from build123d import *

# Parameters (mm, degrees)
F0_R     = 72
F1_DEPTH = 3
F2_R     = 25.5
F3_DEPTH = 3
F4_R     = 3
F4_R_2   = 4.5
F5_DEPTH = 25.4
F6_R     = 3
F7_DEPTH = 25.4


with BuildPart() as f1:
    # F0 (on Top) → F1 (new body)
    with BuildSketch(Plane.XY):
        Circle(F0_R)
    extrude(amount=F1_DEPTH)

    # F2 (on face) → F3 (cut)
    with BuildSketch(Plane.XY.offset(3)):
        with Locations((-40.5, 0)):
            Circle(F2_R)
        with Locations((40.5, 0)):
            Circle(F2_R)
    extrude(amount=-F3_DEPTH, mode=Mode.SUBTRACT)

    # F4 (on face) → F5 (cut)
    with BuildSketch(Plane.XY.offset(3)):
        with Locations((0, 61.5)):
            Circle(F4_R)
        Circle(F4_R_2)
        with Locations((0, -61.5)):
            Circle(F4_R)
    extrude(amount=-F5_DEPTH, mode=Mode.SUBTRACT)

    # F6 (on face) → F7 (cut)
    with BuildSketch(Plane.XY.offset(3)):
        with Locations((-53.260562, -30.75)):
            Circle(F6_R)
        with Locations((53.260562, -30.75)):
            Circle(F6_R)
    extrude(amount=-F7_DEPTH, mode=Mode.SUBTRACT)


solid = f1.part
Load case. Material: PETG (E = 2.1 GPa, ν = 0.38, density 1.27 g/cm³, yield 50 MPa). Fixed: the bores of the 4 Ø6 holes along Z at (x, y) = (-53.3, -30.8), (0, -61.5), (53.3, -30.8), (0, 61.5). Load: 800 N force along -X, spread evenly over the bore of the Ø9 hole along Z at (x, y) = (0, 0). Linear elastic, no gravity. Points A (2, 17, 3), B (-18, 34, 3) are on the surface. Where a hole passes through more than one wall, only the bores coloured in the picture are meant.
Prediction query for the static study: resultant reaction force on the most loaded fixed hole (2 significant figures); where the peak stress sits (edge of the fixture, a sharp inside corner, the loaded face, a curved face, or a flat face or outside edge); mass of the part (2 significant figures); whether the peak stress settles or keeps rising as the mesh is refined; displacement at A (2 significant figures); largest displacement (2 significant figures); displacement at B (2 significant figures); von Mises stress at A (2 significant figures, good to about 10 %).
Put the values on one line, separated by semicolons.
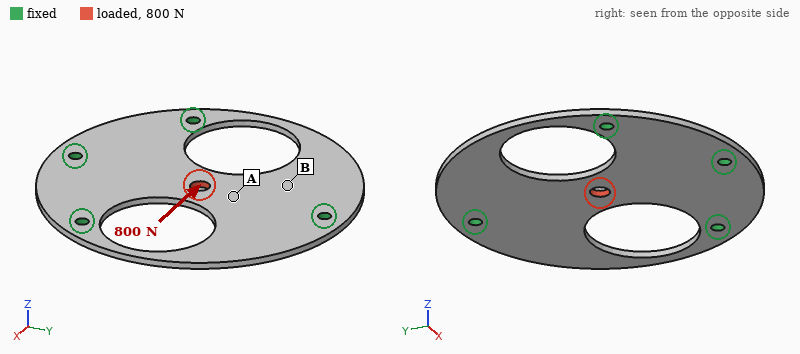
240 N; edge of the fixture; 46 g; keeps rising; 0.28 mm; 0.38 mm; 0.19 mm; 4.8 MPa
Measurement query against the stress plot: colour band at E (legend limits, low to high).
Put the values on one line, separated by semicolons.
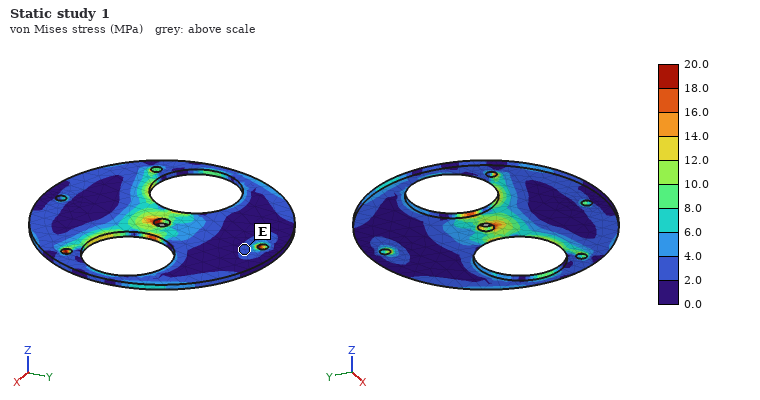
2.0 to 4.0 MPa
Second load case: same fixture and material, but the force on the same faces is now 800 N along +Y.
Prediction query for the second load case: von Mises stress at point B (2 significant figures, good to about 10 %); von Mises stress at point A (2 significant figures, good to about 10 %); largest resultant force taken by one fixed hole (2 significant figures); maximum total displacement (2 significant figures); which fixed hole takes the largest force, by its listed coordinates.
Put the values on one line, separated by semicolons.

1.8 MPa; 4.7 MPa; 340 N; 0.13 mm; (0, 61.5)
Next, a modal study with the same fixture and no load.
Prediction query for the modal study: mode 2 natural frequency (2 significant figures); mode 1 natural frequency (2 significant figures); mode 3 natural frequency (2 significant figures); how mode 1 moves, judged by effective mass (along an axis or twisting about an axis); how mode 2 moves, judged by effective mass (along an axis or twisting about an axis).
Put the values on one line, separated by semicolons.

250 Hz; 220 Hz; 360 Hz; twisting about Y; along Z
